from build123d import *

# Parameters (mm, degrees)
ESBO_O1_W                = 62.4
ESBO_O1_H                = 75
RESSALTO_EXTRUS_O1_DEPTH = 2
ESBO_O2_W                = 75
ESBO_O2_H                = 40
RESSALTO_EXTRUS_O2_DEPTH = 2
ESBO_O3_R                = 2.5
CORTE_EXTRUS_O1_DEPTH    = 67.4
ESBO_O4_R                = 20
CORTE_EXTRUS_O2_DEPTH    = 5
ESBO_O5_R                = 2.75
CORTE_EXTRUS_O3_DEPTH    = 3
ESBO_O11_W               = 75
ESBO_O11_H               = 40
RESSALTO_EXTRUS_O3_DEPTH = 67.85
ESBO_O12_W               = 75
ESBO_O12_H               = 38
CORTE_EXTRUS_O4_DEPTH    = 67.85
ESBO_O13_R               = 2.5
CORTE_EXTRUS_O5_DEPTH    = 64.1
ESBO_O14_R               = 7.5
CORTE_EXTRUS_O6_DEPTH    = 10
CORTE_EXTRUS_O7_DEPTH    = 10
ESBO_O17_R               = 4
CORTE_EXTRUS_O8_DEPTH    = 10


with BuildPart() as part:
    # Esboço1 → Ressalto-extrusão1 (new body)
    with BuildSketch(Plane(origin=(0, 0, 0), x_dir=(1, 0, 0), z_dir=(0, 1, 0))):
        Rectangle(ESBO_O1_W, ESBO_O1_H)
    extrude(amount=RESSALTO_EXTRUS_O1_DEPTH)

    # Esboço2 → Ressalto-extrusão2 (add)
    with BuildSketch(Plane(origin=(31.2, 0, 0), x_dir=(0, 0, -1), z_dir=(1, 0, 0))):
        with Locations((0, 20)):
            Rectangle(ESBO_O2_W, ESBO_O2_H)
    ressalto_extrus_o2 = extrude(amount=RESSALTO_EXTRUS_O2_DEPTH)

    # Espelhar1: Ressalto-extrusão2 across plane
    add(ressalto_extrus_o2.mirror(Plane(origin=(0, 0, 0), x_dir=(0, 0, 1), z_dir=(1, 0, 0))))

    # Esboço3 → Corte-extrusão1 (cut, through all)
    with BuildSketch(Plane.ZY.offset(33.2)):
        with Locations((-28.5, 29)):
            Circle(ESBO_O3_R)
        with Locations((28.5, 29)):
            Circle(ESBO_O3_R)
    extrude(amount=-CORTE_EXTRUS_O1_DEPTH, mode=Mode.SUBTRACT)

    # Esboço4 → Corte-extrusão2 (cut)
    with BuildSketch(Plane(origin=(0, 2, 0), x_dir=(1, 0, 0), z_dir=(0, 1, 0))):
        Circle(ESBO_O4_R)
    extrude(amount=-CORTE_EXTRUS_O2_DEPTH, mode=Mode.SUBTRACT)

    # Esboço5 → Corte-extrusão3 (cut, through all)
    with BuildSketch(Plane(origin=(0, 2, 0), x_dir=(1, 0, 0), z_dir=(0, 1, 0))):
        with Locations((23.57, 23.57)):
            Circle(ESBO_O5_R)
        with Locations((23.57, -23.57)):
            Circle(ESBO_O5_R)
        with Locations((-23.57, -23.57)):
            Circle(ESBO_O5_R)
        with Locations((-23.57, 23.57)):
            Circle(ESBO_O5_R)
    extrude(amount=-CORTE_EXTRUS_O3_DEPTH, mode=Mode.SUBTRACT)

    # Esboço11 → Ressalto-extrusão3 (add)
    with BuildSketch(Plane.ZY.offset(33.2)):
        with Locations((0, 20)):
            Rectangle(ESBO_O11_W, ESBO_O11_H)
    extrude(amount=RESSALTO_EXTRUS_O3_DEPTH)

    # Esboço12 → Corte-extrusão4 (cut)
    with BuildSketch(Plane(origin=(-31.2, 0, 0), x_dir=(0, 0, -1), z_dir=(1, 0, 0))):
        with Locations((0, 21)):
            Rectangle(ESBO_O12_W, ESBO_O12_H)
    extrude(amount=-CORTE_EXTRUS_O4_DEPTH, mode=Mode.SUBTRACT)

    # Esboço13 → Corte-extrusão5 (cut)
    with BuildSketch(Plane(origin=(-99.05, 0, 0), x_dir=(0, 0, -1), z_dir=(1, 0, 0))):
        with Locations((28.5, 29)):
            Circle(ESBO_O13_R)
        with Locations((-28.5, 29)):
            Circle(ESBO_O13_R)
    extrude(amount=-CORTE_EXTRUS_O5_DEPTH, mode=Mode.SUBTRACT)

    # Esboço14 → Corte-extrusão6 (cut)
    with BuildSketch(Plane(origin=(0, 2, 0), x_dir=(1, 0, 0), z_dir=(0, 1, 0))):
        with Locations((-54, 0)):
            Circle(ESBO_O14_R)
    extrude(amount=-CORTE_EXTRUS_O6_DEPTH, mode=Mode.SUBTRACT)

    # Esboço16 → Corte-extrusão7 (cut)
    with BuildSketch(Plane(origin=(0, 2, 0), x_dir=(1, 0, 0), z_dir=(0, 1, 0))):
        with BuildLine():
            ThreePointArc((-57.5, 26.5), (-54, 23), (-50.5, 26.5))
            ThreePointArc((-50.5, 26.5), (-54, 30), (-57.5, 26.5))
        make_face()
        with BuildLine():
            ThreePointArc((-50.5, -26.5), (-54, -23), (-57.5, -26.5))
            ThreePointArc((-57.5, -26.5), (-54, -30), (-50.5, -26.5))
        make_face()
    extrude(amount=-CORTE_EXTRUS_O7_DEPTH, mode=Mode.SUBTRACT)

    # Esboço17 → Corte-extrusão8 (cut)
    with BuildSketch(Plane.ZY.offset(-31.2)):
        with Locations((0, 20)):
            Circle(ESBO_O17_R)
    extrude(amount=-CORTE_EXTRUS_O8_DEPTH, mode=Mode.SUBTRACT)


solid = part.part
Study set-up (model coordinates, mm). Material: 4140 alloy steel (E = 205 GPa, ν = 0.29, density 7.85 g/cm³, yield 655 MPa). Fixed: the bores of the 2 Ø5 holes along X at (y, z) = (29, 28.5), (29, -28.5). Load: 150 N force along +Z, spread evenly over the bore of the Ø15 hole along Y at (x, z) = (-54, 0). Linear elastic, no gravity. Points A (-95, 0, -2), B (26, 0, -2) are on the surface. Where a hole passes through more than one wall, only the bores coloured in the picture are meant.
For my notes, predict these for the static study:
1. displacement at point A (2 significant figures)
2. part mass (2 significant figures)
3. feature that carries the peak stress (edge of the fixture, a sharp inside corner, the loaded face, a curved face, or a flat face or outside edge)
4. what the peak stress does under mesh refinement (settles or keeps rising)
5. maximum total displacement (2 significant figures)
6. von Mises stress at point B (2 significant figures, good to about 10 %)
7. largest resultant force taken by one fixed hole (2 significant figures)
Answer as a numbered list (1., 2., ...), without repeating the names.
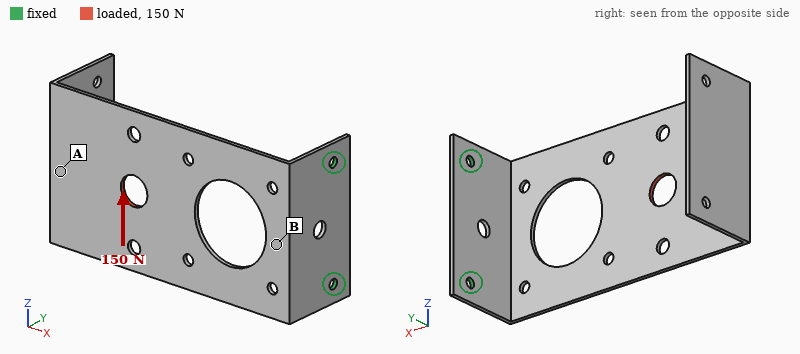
1. 0.85 mm
2. 220 g
3. edge of the fixture
4. keeps rising
5. 1.2 mm
6. 57 MPa
7. 240 N
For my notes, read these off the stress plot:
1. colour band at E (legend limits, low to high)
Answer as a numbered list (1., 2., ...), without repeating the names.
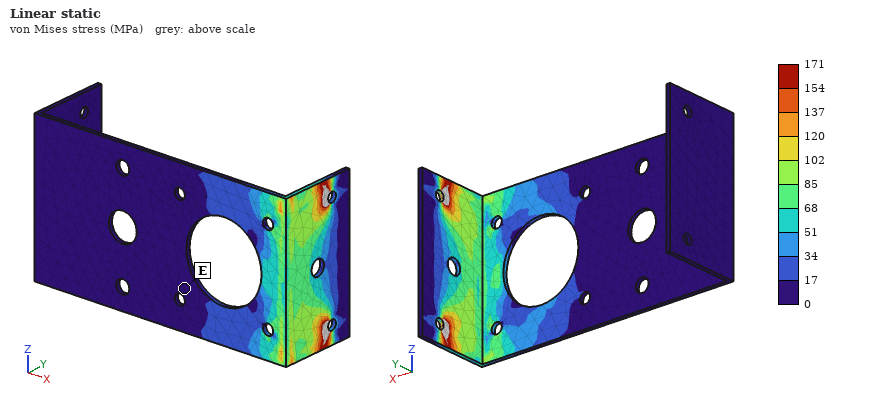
1. 0 to 17 MPa
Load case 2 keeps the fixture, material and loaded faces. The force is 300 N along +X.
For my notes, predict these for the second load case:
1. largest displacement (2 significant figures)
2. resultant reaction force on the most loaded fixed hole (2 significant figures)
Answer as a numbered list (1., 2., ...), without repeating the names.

1. 1.7 mm
2. 150 N
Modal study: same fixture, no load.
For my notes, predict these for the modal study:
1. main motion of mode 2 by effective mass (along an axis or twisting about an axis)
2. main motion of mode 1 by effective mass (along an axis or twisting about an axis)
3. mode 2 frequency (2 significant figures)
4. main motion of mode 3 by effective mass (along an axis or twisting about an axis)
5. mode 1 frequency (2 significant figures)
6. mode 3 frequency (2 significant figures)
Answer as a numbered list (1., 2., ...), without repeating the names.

1. along Z
2. along Y
3. 140 Hz
4. along Z
5. 42 Hz
6. 260 Hz
